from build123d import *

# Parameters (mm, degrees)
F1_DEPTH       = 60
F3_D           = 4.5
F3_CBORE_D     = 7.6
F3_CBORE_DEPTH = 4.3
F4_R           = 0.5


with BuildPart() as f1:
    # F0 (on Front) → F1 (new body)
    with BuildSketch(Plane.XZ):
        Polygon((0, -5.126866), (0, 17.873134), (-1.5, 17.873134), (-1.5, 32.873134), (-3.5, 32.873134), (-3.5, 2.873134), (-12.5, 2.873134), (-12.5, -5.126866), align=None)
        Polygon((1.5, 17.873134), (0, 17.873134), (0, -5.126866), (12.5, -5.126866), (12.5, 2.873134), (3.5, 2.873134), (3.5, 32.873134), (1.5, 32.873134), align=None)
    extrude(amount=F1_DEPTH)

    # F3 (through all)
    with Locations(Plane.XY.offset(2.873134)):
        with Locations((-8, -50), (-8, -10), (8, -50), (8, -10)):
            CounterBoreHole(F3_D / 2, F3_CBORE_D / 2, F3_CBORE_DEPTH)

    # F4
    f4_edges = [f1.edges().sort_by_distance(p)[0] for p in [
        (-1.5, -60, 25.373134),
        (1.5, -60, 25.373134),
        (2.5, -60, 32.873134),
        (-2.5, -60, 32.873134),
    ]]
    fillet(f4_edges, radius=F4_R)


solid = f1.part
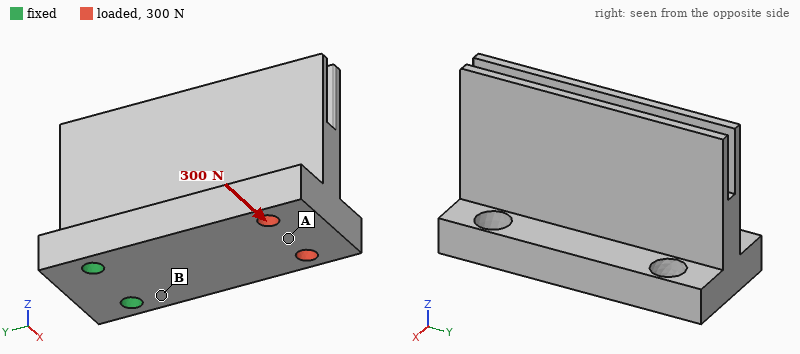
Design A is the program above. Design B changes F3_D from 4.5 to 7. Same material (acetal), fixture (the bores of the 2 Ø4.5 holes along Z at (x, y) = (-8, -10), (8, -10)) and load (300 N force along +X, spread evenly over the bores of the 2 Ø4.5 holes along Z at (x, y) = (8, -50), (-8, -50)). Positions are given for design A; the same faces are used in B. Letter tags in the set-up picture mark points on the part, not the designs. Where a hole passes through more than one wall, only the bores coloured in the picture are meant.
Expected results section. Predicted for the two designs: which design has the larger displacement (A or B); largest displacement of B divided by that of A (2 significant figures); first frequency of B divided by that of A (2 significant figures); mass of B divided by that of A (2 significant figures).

A
0.87
1.4
0.98
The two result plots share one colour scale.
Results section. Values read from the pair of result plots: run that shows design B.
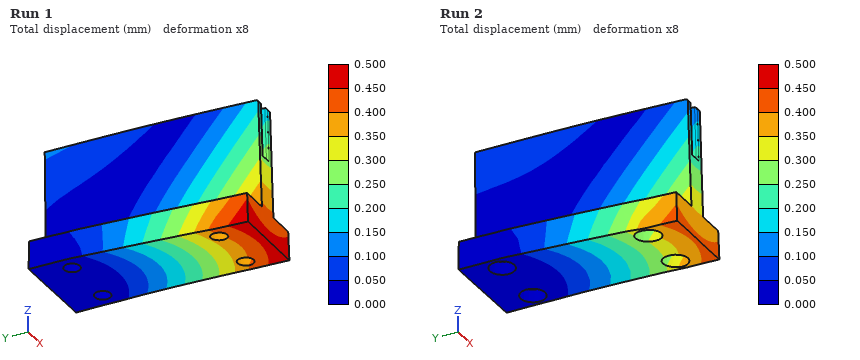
Run 2
